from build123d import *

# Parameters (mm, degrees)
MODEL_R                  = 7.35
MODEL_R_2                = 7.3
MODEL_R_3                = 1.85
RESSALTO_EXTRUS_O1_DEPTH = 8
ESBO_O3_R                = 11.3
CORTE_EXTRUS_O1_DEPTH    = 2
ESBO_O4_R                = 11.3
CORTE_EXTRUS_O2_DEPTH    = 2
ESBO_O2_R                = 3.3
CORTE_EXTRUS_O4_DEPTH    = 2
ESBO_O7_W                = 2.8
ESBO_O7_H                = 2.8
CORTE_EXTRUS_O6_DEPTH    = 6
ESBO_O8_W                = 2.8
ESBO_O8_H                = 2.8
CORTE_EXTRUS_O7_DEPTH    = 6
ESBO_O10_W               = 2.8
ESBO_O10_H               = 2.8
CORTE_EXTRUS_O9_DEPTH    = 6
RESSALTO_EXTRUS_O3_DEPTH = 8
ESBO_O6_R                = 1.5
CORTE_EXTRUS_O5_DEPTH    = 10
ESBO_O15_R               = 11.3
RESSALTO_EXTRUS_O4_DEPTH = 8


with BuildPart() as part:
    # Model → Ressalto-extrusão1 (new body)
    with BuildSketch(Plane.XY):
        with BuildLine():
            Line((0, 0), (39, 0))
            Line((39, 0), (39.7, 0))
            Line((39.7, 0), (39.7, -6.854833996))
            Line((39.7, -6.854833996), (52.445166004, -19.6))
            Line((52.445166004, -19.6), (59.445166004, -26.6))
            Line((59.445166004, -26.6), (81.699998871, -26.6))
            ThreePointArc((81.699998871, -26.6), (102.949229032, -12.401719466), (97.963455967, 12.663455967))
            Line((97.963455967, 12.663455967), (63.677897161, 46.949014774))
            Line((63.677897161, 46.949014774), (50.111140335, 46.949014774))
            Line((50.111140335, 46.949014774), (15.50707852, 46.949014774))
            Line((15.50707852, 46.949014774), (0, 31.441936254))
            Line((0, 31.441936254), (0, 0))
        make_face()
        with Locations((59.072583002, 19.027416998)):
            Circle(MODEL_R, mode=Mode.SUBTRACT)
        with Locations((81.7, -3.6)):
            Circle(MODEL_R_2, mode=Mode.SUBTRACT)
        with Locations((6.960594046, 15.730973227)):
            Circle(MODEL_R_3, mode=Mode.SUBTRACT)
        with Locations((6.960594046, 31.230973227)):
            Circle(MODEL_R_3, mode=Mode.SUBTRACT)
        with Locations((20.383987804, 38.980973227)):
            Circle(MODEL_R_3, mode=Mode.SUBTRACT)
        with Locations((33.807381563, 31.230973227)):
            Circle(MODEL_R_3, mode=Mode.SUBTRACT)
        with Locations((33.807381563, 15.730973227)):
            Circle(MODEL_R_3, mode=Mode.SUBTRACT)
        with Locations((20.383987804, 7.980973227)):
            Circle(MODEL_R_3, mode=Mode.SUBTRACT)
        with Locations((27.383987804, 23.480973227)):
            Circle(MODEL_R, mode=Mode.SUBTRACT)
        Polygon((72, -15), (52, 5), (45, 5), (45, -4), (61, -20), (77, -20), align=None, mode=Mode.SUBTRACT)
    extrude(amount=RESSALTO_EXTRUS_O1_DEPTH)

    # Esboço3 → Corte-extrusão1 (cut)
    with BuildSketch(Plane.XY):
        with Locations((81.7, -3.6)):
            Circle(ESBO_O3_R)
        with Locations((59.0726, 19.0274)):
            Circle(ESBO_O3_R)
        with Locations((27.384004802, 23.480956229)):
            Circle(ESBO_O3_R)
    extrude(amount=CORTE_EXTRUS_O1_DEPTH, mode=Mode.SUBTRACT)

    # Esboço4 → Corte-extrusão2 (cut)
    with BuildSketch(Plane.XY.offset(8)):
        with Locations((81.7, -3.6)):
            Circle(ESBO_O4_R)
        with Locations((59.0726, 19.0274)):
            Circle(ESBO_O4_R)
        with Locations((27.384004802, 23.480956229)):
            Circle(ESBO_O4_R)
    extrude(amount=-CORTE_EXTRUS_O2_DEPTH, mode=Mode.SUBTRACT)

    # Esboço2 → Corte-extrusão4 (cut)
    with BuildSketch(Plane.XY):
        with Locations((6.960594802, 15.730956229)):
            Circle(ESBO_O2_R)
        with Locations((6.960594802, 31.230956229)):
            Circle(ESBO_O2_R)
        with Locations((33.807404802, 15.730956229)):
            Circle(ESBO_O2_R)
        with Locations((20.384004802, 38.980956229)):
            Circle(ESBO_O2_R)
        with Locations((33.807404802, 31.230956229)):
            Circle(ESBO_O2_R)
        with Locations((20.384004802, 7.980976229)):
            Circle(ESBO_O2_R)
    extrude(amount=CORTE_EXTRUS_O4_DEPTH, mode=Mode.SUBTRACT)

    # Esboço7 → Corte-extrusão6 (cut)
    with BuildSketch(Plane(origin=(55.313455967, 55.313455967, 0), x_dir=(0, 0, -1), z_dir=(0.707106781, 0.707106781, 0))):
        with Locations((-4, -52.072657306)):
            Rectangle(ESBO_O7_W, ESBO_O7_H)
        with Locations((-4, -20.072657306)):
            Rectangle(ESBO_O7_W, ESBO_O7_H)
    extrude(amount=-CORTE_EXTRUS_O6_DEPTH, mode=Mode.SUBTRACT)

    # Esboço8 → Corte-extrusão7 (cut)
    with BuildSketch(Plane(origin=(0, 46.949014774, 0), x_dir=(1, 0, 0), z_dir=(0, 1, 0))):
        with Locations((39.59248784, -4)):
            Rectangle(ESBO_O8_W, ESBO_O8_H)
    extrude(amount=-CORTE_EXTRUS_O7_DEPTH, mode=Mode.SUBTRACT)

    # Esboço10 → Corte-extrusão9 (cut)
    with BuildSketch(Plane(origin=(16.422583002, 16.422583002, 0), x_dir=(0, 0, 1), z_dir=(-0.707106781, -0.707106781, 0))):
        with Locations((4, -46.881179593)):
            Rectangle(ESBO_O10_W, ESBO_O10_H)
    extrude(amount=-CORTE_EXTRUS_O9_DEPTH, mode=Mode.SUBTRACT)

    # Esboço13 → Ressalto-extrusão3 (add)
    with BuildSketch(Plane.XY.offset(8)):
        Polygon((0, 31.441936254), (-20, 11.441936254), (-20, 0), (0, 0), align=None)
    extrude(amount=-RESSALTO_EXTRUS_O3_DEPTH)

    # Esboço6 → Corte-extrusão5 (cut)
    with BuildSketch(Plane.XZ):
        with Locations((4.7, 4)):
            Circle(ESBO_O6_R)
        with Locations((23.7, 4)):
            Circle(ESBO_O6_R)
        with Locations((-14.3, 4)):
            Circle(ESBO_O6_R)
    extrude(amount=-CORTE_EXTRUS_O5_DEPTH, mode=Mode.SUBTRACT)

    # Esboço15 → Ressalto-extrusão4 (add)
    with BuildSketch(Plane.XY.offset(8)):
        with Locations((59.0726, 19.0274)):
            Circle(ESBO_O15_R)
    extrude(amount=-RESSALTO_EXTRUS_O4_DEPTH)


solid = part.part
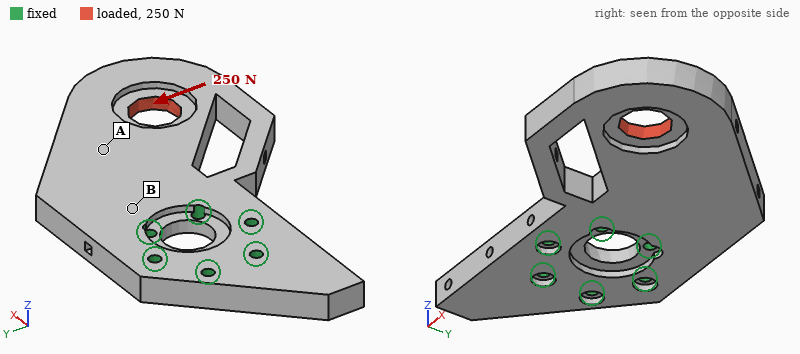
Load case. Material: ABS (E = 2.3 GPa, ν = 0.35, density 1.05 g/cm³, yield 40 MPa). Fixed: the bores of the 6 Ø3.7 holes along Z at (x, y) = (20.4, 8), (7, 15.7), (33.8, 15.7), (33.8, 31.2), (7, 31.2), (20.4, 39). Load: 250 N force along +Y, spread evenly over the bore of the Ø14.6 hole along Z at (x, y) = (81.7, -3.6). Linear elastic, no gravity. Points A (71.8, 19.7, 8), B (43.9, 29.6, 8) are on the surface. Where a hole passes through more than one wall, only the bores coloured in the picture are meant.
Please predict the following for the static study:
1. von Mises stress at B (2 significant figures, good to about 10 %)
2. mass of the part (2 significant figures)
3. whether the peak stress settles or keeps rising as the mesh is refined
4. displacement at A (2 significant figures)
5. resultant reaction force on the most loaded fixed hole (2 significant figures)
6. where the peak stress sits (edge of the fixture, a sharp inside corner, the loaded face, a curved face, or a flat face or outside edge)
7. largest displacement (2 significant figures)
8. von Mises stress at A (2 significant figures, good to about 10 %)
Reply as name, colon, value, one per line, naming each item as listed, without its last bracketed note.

von Mises stress at B: 2.8 MPa
mass of the part: 40 g
whether the peak stress settles or keeps rising as the mesh is refined: keeps rising
displacement at A: 0.13 mm
resultant reaction force on the most loaded fixed hole: 280 N
where the peak stress sits: edge of the fixture
largest displacement: 0.30 mm
von Mises stress at A: 1.4 MPa
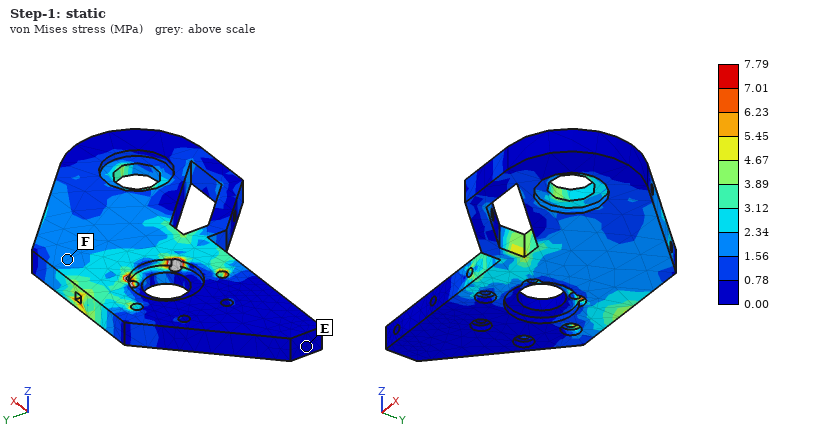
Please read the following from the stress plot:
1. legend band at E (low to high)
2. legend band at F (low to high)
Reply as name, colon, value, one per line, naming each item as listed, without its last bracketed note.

legend band at E: 0.00 to 0.78 MPa
legend band at F: 1.56 to 2.34 MPa
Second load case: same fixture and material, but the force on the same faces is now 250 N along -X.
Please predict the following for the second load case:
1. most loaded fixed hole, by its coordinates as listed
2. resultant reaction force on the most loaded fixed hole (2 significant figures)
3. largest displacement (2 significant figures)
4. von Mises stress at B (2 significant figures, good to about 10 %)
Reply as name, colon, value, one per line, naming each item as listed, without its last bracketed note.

most loaded fixed hole, by its coordinates as listed: (33.8, 15.7)
resultant reaction force on the most loaded fixed hole: 230 N
largest displacement: 0.22 mm
von Mises stress at B: 0.60 MPa
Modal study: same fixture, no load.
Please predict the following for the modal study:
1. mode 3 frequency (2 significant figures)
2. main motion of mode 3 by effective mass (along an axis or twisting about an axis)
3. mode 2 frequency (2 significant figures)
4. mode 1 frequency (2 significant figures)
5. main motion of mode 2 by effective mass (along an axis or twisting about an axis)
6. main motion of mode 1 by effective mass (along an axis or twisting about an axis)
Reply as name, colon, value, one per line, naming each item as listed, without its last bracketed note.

mode 3 frequency: 1300 Hz
main motion of mode 3 by effective mass: along Y
mode 2 frequency: 870 Hz
mode 1 frequency: 330 Hz
main motion of mode 2 by effective mass: twisting about X
main motion of mode 1 by effective mass: along Z
